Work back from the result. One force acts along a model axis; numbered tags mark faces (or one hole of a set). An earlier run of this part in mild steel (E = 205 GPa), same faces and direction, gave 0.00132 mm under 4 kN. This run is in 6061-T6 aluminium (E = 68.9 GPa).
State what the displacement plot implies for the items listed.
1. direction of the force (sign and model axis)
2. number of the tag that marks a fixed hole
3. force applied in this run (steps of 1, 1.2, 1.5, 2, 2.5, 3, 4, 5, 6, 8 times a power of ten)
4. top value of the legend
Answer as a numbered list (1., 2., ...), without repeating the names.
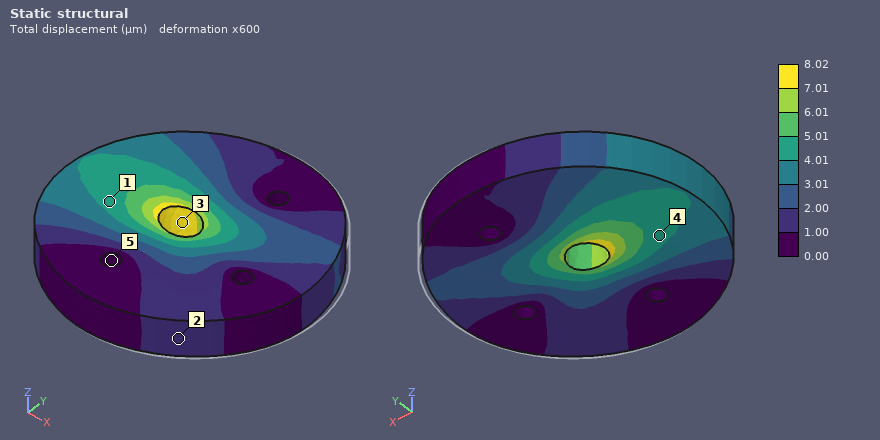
1. -X
2. 5
3. 8 kN
4. 8.02 µm
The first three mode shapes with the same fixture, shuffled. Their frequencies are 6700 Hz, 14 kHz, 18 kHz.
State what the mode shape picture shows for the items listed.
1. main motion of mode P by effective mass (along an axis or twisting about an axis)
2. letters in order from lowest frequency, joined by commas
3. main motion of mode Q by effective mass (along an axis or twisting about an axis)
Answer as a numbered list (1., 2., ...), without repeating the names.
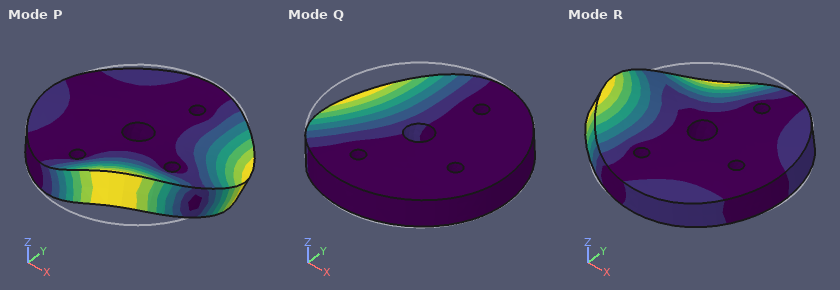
1. twisting about X
2. Q, R, P
3. along Z
